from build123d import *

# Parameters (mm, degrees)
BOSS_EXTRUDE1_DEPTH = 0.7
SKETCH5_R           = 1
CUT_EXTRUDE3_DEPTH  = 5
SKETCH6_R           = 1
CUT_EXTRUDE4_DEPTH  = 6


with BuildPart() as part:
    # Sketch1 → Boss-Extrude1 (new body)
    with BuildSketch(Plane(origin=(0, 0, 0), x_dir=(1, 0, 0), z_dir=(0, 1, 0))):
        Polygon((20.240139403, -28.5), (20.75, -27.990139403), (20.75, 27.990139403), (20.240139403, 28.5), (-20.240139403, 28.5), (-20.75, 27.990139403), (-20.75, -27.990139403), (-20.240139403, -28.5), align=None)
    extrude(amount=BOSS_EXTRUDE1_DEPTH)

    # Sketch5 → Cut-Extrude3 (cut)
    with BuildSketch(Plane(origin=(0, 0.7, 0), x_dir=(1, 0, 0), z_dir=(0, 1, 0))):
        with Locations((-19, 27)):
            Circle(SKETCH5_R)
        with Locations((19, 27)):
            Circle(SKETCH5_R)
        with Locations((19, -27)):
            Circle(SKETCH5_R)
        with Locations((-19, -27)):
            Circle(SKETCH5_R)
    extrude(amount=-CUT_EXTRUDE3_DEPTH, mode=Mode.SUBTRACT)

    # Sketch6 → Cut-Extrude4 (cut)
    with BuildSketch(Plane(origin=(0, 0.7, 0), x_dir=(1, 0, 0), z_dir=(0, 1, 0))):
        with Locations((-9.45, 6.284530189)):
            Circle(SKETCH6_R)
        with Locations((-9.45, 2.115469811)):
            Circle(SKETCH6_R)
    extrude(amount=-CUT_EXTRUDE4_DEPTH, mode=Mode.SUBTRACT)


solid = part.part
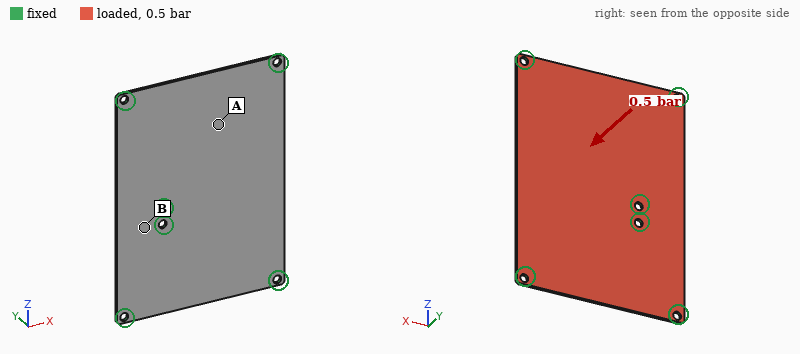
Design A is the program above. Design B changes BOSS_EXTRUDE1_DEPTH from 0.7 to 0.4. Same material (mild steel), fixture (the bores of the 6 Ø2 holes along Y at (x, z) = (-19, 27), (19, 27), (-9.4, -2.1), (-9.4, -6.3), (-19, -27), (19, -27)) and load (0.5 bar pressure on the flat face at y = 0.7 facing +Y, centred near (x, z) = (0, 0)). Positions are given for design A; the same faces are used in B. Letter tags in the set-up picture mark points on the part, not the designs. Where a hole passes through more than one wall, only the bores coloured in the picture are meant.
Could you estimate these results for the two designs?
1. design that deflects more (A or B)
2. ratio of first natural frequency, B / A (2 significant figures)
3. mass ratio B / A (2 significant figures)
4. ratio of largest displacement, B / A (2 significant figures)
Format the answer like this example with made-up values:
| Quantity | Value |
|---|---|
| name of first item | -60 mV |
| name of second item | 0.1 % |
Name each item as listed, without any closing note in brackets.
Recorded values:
| Quantity | Value |
|---|---|
| design that deflects more | B |
| ratio of first natural frequency, B / A | 0.58 |
| mass ratio B / A | 0.57 |
| ratio of largest displacement, B / A | 5.3 |
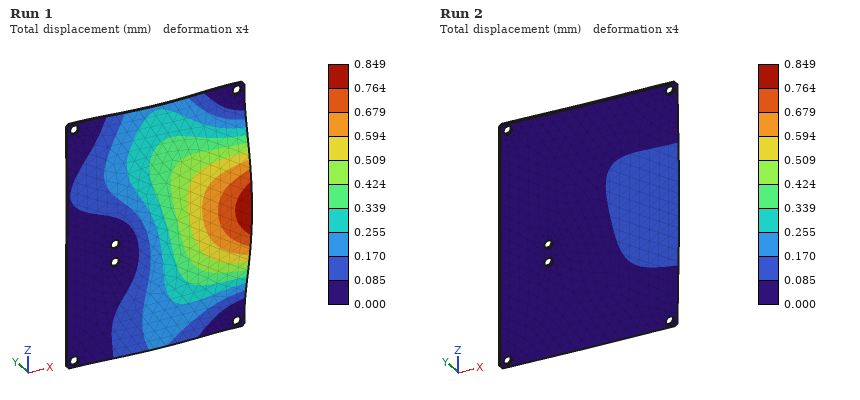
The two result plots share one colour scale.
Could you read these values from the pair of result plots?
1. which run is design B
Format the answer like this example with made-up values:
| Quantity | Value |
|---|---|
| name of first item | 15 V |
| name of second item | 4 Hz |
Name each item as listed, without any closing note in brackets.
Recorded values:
| Quantity | Value |
|---|---|
| which run is design B | Run 1 |
